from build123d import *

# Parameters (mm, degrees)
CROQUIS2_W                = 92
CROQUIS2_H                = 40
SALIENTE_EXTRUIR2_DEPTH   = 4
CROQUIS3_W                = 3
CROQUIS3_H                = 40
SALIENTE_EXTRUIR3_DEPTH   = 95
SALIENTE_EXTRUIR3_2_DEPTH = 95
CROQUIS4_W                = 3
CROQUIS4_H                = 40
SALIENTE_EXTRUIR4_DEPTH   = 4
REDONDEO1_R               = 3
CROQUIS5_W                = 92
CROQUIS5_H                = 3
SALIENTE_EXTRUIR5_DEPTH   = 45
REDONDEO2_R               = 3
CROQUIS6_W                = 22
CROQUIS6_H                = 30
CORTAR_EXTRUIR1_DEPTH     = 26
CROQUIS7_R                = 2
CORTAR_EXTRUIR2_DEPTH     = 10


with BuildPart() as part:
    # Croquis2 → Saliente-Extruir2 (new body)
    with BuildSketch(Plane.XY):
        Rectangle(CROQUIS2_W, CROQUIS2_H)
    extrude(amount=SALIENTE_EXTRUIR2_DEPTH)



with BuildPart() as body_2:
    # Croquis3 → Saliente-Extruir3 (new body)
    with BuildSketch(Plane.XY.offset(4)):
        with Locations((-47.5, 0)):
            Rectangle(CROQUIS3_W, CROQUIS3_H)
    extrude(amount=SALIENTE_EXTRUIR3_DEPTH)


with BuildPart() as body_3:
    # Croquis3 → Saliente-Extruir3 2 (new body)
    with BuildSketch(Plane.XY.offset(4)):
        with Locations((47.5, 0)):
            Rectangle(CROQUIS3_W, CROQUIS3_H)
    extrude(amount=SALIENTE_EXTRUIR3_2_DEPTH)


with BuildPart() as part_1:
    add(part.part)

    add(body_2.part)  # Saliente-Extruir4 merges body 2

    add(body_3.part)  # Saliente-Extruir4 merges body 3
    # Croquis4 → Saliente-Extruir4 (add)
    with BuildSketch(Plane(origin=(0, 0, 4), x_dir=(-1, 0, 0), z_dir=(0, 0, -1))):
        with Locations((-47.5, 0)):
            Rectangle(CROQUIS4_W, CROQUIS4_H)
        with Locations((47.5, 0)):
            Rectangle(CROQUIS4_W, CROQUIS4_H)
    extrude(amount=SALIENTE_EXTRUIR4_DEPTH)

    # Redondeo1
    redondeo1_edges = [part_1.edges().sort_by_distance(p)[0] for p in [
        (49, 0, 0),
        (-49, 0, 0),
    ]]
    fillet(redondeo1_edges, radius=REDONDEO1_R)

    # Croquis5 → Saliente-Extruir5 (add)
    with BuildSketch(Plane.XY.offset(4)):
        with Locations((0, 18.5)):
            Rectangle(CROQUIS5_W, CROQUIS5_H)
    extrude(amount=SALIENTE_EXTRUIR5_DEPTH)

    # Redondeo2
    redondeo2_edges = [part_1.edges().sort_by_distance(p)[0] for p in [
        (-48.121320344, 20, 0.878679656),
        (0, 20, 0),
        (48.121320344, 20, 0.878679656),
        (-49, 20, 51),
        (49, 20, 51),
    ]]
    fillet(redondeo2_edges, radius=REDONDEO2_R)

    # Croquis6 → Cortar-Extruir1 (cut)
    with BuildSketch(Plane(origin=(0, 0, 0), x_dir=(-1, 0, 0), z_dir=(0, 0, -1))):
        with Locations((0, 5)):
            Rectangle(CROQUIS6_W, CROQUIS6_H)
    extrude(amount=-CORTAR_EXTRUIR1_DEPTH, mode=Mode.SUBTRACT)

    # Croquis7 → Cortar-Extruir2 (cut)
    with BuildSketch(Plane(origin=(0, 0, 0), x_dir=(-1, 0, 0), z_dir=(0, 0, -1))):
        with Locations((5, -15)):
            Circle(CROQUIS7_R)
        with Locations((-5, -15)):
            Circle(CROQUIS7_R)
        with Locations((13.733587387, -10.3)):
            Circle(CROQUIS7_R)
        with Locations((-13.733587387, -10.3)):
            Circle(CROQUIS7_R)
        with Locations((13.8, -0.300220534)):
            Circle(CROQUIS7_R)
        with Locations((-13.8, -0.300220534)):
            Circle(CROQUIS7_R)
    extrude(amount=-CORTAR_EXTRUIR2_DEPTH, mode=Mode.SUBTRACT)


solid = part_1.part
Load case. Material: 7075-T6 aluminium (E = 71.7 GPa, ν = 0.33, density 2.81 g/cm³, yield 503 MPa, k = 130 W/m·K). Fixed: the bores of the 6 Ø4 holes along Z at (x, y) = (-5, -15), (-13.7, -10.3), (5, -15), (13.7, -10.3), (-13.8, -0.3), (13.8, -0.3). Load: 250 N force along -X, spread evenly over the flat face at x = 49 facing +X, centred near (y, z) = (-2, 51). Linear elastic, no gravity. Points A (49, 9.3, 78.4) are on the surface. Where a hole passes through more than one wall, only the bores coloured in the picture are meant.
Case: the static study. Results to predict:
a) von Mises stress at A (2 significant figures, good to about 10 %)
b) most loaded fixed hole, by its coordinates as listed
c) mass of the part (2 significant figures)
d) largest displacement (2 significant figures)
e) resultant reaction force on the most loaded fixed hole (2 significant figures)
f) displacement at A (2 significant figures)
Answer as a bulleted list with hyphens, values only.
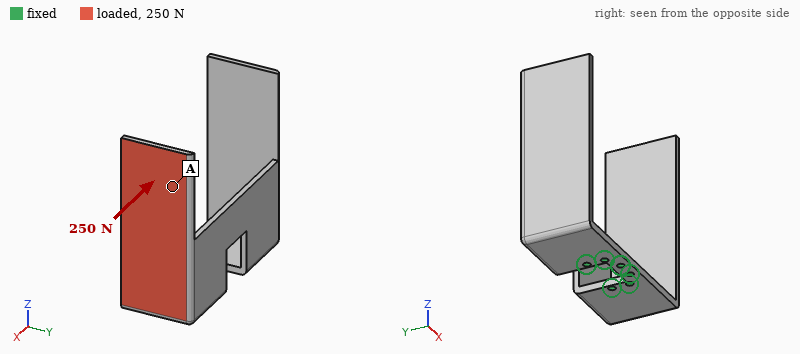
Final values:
- 13 MPa
- (-13.8, -0.3)
- 130 g
- 1.7 mm
- 440 N
- 0.82 mm
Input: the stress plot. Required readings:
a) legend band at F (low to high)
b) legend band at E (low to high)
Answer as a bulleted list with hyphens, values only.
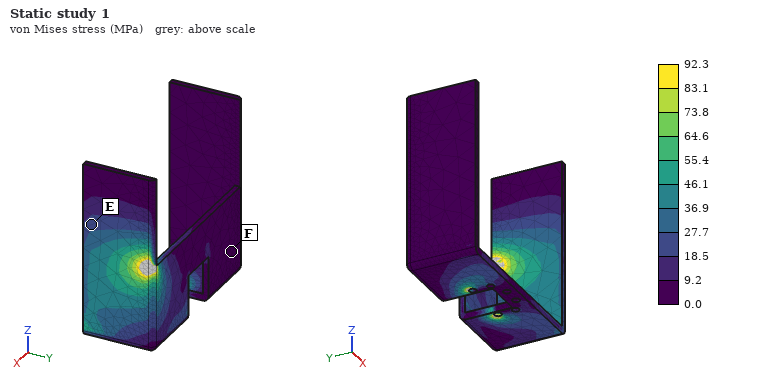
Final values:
- 0.0 to 9.2 MPa
- 18.5 to 27.7 MPa
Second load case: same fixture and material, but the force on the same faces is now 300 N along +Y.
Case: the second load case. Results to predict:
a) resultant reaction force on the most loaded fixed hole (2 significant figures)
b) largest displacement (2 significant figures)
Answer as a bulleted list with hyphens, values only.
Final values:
- 970 N
- 1.4 mm
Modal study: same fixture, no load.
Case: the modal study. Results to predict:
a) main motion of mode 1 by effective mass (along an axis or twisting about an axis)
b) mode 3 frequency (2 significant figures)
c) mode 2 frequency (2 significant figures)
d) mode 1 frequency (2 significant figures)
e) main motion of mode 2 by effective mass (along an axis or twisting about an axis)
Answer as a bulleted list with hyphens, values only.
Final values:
- along X
- 540 Hz
- 460 Hz
- 380 Hz
- along Y
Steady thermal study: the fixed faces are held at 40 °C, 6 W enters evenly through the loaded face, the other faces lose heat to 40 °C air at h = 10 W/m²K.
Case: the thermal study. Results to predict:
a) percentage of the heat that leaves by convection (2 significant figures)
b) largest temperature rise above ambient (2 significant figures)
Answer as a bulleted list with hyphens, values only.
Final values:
- 20 %
- 18 K
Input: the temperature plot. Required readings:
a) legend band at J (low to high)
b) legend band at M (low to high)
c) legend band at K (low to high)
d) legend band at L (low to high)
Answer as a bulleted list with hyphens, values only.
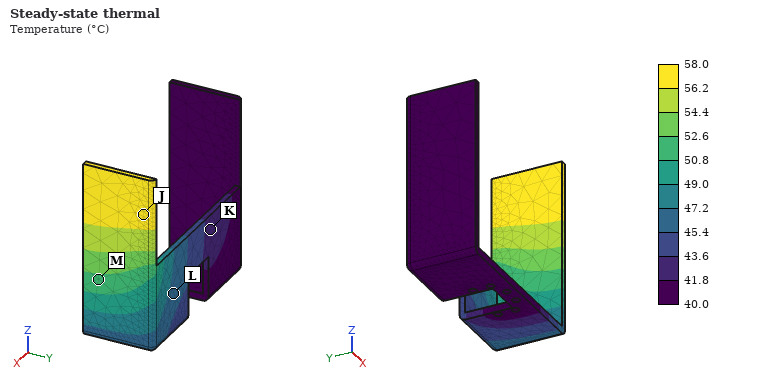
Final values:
- 56.2 to 58.0 °C
- 50.8 to 52.6 °C
- 41.8 to 43.6 °C
- 45.4 to 47.2 °C
